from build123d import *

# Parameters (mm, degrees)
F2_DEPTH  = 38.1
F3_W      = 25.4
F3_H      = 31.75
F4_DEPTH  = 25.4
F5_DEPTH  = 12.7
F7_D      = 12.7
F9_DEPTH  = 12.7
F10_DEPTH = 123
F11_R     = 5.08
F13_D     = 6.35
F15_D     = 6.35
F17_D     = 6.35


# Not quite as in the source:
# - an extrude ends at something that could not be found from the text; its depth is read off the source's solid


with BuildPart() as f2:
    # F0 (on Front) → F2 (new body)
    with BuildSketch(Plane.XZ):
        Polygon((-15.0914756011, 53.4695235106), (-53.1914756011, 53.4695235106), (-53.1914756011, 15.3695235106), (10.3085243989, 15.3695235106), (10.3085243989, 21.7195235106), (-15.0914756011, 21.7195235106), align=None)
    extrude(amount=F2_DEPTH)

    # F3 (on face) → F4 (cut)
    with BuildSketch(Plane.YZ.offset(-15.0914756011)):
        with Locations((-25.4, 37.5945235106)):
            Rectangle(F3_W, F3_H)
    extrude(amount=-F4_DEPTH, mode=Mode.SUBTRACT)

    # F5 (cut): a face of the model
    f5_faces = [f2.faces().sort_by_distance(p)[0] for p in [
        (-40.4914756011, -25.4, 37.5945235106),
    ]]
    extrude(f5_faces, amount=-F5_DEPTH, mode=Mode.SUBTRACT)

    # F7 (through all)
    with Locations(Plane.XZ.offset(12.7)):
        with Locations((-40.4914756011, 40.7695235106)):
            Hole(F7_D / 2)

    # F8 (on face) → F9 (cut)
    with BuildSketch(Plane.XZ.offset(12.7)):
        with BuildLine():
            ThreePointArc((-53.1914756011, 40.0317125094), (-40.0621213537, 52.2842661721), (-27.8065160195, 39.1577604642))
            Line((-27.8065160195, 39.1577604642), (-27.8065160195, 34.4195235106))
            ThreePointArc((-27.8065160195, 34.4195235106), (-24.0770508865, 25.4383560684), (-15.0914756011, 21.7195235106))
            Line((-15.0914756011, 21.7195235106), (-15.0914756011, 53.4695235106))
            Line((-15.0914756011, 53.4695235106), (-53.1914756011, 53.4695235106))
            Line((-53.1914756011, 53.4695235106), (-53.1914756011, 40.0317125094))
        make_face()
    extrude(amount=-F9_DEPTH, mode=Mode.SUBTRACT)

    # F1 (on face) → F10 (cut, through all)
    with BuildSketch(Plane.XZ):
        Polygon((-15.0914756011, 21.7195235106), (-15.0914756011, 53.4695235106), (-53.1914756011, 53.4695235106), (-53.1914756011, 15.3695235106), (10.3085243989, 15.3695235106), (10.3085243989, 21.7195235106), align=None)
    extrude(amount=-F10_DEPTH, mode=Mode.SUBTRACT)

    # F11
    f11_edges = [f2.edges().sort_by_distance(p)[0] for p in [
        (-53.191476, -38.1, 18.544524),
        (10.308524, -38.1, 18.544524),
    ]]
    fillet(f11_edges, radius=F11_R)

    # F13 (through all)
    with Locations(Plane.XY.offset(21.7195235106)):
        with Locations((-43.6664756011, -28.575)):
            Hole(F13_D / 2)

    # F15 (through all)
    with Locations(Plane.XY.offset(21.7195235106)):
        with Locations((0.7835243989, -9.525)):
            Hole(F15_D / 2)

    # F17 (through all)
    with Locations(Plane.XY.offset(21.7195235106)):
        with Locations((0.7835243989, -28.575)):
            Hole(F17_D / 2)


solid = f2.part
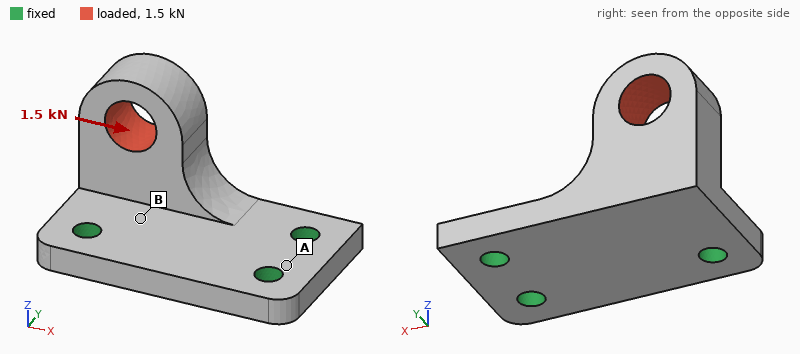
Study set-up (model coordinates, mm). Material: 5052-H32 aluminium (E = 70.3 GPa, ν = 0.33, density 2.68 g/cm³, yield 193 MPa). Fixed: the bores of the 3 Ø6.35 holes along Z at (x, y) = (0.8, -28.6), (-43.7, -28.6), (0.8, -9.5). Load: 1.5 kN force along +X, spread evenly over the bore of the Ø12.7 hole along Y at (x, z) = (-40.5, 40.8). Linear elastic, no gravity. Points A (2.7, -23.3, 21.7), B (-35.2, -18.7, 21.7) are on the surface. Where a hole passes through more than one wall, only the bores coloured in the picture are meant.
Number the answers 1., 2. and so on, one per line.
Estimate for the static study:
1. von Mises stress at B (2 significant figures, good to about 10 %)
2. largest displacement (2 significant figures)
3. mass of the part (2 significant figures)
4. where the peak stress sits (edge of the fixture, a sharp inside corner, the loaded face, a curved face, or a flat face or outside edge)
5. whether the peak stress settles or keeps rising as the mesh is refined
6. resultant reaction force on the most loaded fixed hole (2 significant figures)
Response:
1. 37 MPa
2. 0.11 mm
3. 60 g
4. edge of the fixture
5. keeps rising
6. 960 N
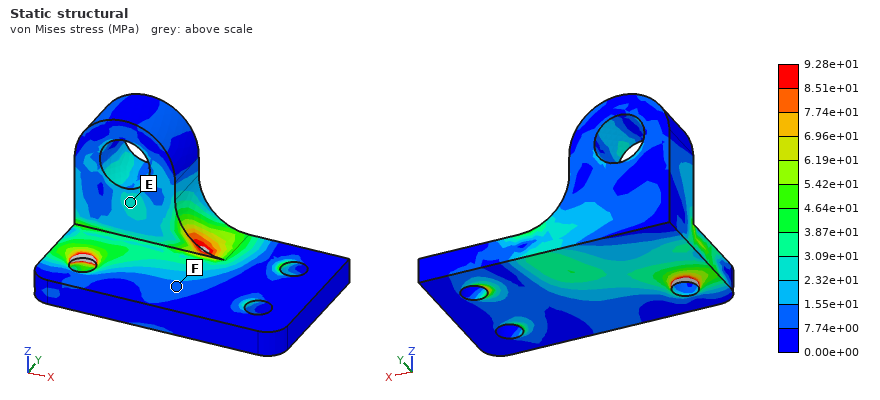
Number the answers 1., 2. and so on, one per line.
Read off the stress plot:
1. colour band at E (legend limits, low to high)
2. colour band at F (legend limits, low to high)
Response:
1. 2.32e+01 to 3.09e+01 MPa
2. 7.74e+00 to 1.55e+01 MPa
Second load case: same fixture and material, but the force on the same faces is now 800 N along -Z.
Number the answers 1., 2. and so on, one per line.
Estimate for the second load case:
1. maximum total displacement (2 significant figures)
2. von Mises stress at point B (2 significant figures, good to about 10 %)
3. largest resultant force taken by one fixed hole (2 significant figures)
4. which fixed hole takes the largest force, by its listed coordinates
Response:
1. 85 µm
2. 22 MPa
3. 650 N
4. (-43.7, -28.6)
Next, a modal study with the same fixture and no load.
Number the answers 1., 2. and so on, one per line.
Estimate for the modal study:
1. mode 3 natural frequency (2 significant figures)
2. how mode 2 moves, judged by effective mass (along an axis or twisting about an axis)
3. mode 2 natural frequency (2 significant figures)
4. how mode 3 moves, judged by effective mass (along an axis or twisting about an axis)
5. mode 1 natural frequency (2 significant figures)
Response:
1. 9300 Hz
2. along X
3. 6800 Hz
4. along Z
5. 3100 Hz
